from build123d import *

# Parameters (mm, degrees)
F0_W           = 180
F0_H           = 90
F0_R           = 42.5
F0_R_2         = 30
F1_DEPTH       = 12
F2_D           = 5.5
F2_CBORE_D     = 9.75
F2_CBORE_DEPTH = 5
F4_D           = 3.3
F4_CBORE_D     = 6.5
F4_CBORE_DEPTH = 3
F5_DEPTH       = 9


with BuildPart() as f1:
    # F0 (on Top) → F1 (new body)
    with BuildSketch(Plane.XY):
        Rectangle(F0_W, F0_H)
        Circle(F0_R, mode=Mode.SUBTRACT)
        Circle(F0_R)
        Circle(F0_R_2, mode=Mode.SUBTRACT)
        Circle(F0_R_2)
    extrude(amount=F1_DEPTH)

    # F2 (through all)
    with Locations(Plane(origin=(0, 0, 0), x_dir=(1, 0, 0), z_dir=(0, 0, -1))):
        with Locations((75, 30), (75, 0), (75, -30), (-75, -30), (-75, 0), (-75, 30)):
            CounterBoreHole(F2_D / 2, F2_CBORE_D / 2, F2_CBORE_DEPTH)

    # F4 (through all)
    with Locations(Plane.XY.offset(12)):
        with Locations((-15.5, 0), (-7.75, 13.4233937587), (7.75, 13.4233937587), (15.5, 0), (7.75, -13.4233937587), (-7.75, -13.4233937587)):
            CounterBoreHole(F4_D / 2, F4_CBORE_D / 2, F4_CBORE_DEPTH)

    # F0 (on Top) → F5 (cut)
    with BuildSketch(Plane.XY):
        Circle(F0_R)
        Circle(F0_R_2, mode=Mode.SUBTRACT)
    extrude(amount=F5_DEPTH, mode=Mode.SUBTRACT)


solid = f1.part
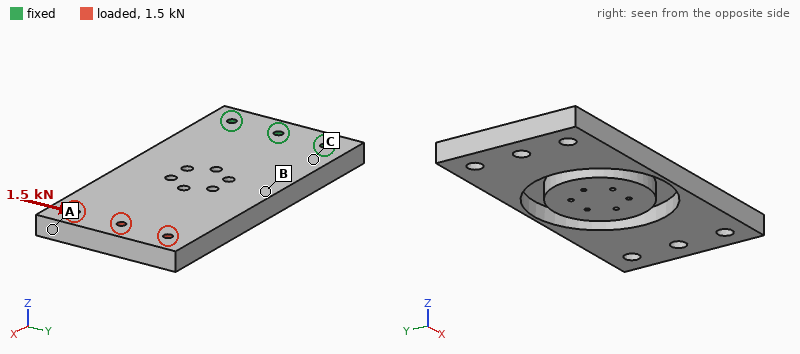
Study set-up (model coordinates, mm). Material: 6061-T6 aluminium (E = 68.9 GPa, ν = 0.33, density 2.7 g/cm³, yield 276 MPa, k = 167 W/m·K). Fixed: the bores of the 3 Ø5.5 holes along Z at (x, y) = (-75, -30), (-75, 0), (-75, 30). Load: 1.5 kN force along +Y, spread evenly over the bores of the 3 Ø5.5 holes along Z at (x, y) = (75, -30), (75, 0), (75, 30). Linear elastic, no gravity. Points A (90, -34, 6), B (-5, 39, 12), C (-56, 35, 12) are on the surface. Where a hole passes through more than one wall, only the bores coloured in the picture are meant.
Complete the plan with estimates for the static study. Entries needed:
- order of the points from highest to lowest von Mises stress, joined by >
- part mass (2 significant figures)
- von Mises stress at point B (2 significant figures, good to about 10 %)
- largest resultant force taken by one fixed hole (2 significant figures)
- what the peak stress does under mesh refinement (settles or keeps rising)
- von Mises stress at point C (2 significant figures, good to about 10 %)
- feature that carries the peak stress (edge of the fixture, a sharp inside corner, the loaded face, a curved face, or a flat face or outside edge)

C > B > A
440 g
12 MPa
3.7 kN
keeps rising
18 MPa
edge of the fixture
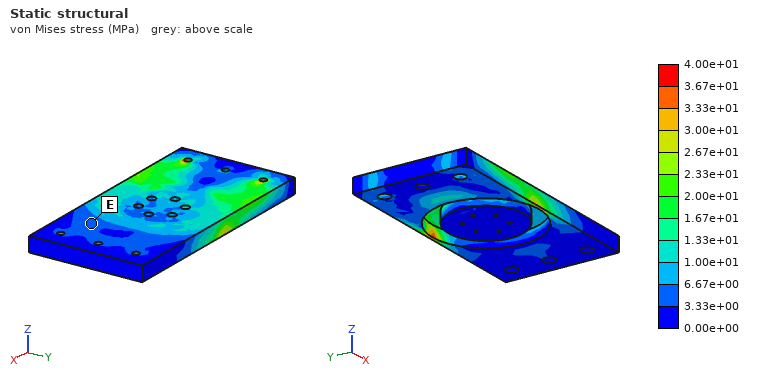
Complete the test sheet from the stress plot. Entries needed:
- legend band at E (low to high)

3.33e+00 to 6.67e+00 MPa
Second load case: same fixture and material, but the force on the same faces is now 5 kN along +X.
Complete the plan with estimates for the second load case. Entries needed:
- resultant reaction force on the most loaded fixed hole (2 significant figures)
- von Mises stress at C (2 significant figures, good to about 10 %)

1.8 kN
11 MPa
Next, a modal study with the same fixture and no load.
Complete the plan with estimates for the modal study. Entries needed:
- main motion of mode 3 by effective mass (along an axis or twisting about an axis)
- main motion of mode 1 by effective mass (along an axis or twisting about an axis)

along Z
along Z
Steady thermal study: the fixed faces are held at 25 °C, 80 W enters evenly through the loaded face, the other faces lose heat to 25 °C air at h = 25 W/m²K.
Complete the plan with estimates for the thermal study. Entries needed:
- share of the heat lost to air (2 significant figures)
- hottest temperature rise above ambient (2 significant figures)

46 %
73 K
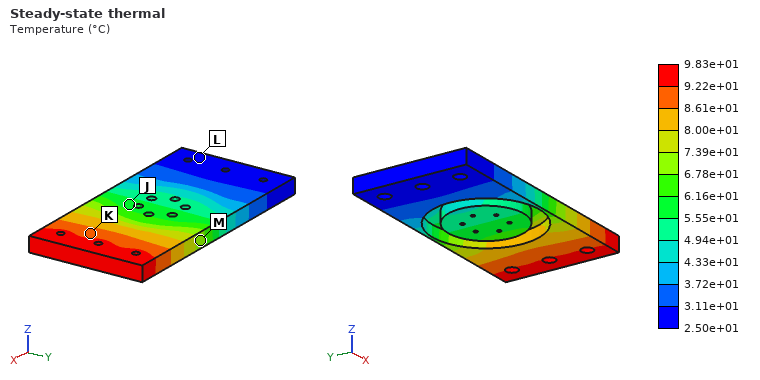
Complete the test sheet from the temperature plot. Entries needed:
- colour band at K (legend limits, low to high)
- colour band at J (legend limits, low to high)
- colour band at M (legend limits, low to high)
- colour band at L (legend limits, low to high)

8.61e+01 to 9.22e+01 °C
5.55e+01 to 6.16e+01 °C
6.78e+01 to 7.39e+01 °C
2.50e+01 to 3.11e+01 °C
